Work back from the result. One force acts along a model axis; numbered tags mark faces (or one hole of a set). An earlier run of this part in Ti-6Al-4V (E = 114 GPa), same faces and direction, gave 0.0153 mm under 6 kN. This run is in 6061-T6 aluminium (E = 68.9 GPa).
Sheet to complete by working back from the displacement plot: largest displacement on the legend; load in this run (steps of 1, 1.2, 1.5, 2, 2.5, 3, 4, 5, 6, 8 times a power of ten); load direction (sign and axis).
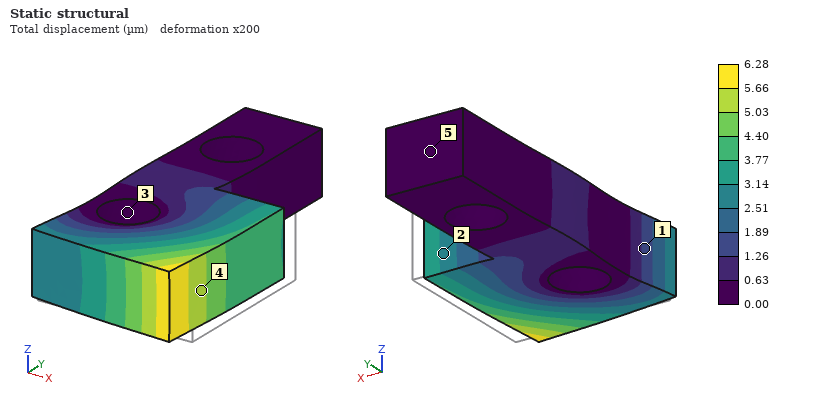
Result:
6.28 µm
1.5 kN
-X
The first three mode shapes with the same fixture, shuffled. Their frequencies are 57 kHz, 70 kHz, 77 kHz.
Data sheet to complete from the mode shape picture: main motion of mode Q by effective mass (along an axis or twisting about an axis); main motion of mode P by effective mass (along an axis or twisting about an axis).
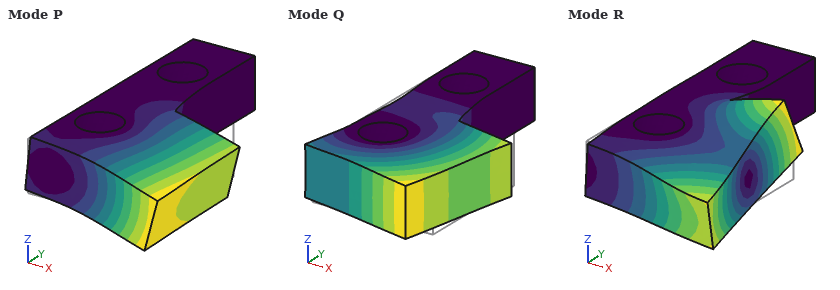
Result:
along Y
along Z
